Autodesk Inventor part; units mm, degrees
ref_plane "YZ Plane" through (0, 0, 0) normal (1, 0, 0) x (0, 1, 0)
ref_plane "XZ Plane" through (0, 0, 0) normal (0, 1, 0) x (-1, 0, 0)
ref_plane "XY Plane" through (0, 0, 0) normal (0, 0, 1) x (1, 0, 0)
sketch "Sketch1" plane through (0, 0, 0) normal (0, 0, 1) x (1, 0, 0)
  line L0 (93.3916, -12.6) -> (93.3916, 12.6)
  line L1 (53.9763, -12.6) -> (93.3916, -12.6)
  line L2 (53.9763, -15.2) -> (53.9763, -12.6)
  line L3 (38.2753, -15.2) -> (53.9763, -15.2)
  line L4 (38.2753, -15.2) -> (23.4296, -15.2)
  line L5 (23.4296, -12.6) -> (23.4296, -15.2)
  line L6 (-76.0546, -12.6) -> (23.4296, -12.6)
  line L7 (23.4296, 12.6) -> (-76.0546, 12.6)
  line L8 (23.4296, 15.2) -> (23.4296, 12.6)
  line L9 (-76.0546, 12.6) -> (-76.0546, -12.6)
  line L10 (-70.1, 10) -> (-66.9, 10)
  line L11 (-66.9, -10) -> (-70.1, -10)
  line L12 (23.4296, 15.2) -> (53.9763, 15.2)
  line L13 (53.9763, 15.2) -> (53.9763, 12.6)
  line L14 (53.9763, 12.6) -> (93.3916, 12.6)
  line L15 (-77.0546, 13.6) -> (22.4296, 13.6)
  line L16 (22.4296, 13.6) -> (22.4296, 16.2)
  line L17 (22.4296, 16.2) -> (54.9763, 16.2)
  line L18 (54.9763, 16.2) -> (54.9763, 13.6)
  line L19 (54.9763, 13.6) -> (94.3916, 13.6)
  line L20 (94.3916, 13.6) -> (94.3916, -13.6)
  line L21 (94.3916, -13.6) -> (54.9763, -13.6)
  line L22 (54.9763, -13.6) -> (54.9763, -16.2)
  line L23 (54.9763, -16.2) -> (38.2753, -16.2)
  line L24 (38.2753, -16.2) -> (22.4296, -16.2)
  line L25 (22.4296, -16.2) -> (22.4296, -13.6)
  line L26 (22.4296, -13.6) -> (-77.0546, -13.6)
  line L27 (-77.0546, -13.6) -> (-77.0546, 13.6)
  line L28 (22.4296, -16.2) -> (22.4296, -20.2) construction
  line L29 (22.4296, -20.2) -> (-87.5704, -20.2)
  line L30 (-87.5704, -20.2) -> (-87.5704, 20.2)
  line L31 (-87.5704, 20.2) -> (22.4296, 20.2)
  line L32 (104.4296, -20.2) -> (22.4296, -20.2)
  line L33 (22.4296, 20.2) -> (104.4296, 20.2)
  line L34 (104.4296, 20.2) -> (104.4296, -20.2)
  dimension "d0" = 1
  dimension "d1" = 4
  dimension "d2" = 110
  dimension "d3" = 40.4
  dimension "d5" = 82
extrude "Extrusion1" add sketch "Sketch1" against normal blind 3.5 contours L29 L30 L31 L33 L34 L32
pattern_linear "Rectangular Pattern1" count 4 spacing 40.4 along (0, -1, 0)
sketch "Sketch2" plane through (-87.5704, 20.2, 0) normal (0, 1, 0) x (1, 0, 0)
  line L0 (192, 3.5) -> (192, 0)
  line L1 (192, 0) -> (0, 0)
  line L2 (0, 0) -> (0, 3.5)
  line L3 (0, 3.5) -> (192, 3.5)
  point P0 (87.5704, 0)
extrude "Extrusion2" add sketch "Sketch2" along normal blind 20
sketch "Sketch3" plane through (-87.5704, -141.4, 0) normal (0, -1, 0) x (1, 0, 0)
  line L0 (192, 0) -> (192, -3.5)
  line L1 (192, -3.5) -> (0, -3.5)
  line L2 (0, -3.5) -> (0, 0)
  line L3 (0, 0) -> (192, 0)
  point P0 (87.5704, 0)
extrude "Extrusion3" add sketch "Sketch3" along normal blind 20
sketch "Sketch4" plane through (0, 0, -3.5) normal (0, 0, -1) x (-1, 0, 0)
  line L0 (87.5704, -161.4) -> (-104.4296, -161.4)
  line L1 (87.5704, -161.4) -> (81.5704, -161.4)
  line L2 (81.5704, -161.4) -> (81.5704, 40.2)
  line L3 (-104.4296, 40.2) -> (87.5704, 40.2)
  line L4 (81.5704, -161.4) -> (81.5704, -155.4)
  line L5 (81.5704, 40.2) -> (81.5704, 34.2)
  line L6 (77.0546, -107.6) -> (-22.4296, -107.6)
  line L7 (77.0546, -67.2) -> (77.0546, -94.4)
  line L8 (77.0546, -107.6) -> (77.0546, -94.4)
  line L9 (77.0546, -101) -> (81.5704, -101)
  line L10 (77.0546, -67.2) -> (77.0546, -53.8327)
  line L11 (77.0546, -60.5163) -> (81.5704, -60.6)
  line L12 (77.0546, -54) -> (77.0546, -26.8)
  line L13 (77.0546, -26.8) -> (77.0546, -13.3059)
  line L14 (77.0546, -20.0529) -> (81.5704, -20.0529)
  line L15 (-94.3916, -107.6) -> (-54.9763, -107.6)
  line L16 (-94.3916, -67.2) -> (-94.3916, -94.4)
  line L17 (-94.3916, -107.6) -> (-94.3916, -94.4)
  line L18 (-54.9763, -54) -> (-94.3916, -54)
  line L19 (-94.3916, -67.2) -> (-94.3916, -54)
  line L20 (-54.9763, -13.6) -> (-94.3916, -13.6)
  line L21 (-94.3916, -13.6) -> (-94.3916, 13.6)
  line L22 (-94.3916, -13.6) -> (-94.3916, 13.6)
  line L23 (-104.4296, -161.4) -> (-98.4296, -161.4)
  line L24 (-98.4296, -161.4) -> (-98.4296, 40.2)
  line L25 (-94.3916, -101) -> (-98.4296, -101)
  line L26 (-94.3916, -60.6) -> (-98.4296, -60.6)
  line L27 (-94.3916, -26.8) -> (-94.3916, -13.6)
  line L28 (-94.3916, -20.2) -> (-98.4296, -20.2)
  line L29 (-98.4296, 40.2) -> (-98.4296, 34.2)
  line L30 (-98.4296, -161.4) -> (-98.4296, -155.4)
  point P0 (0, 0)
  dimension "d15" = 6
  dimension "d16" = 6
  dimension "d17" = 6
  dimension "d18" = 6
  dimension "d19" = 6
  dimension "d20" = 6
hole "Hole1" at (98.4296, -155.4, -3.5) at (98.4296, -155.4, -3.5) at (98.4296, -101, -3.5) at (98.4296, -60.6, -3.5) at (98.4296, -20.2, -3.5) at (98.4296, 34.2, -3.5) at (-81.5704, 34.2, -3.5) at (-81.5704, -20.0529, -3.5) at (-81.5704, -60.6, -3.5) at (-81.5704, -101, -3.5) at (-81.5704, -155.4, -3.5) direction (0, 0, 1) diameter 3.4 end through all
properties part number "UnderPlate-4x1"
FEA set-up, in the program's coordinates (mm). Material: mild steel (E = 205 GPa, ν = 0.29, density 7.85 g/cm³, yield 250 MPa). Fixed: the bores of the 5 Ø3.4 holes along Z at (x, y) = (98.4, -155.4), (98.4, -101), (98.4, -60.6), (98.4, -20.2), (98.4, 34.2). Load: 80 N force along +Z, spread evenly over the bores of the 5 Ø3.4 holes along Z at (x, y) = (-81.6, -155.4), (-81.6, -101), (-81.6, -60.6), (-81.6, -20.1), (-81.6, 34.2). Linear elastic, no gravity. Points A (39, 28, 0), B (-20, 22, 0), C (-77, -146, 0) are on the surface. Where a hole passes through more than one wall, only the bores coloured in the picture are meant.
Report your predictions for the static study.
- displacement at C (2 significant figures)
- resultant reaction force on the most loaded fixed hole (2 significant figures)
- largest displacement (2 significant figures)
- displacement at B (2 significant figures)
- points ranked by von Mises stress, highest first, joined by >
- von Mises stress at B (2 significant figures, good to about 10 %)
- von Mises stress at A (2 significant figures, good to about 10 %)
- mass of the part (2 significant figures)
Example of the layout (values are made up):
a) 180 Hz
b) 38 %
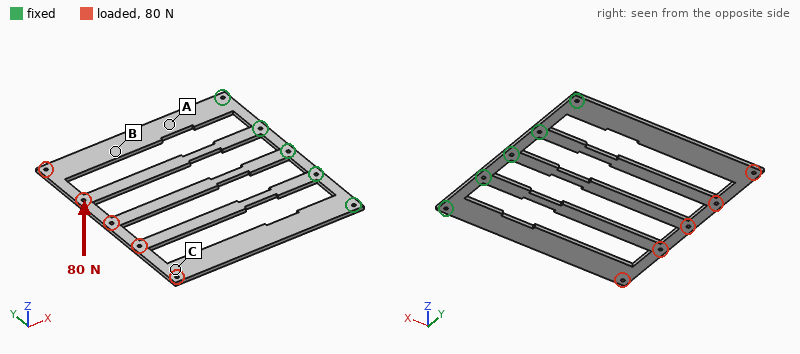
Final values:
a) 2.4 mm
b) 28 N
c) 2.7 mm
d) 1.3 mm
e) A > B > C
f) 28 MPa
g) 58 MPa
h) 530 g
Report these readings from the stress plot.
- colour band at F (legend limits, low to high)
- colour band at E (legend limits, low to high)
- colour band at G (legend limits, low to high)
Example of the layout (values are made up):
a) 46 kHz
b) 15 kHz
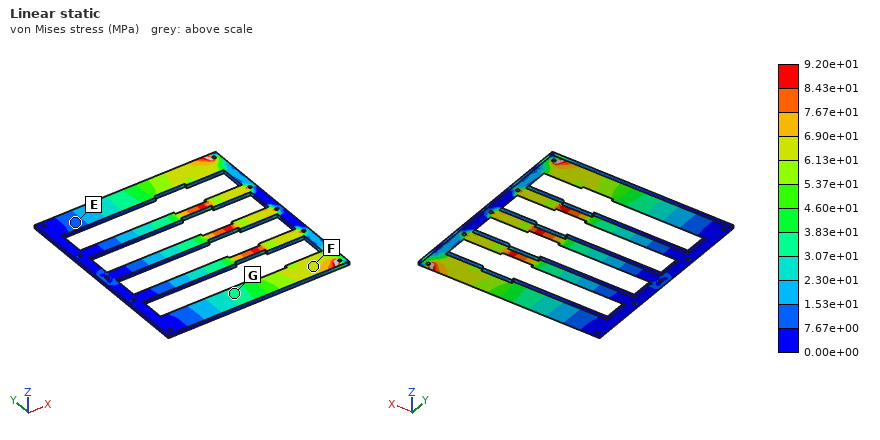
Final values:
a) 6.13e+01 to 6.90e+01 MPa
b) 7.67e+00 to 1.53e+01 MPa
c) 3.07e+01 to 3.83e+01 MPa
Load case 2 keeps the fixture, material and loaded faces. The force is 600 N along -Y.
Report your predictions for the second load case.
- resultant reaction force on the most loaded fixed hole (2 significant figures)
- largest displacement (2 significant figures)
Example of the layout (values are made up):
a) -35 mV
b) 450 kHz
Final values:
a) 760 N
b) 0.28 mm
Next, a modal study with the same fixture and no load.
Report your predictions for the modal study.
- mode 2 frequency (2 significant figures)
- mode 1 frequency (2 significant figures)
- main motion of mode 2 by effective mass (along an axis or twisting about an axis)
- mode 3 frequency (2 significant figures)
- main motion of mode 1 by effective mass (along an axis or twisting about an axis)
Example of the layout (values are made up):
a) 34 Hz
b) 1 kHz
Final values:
a) 150 Hz
b) 71 Hz
c) twisting about X
d) 330 Hz
e) along Z
